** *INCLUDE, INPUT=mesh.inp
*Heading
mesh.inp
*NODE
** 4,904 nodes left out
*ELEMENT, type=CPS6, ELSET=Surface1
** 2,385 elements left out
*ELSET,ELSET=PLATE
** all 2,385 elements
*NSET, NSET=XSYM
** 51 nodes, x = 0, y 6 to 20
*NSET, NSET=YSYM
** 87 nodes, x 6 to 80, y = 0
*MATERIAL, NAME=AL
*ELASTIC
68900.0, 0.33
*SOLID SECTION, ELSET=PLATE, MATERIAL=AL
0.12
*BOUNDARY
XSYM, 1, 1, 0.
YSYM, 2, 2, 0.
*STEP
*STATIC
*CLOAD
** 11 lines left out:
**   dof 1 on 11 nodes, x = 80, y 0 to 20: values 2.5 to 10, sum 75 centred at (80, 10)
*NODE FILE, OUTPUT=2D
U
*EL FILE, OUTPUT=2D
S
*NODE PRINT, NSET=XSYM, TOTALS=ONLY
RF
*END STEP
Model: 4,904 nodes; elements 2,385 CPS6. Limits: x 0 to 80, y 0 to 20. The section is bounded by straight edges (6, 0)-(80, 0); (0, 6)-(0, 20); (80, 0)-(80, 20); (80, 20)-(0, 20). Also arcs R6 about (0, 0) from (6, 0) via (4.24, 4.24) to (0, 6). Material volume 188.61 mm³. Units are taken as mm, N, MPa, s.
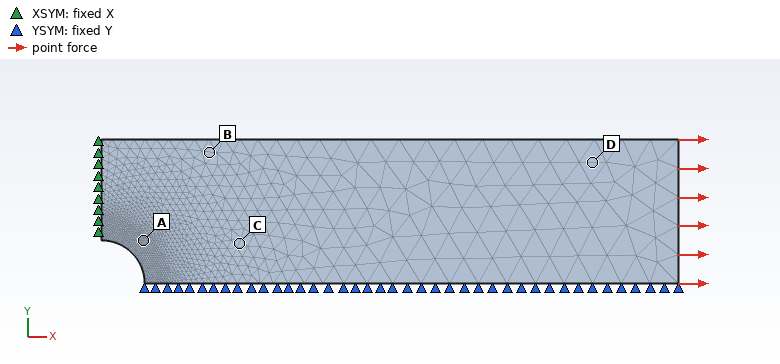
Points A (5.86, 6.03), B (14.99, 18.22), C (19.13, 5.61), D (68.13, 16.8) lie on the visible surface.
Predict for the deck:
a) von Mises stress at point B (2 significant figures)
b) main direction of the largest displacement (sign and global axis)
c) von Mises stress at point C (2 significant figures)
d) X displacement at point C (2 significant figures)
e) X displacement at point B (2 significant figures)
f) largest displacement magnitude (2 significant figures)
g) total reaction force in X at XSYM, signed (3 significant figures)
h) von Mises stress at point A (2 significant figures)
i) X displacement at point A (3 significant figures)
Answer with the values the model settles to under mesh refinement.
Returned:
38 MPa
+X
28 MPa
0.011 mm
0.0077 mm
0.040 mm
-75.0 N
44 MPa
0.00545 mm
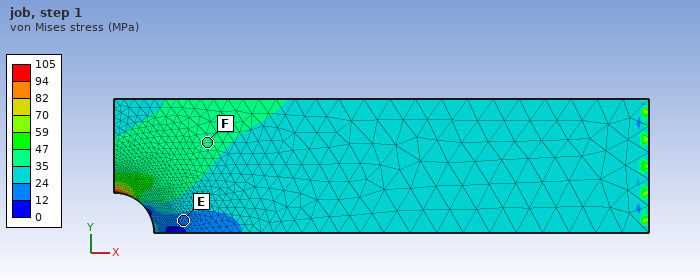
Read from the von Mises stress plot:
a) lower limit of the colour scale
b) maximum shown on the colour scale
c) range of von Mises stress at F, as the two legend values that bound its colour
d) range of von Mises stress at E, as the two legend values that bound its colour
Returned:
0 MPa
105 MPa
35 to 47 MPa
12 to 24 MPa
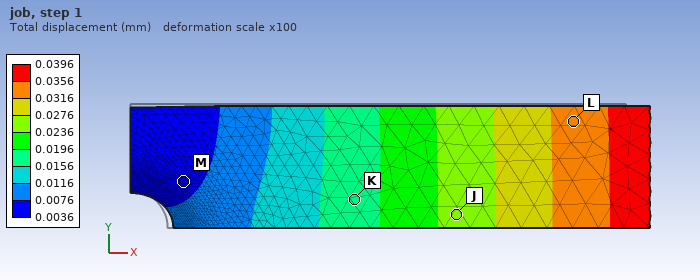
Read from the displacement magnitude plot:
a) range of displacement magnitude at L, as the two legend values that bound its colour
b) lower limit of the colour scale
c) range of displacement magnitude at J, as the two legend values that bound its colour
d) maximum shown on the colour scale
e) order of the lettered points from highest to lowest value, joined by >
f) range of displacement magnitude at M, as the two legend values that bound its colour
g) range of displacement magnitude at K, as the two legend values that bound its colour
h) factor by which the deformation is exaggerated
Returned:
0.0316 to 0.0356 mm
0.0036 mm
0.0236 to 0.0276 mm
0.0396 mm
L > J > K > M
0.0036 to 0.0076 mm
0.0156 to 0.0196 mm
100
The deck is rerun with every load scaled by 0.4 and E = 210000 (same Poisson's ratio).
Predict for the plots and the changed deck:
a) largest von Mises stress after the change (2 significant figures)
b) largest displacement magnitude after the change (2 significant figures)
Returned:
42 MPa
0.0052 mm
